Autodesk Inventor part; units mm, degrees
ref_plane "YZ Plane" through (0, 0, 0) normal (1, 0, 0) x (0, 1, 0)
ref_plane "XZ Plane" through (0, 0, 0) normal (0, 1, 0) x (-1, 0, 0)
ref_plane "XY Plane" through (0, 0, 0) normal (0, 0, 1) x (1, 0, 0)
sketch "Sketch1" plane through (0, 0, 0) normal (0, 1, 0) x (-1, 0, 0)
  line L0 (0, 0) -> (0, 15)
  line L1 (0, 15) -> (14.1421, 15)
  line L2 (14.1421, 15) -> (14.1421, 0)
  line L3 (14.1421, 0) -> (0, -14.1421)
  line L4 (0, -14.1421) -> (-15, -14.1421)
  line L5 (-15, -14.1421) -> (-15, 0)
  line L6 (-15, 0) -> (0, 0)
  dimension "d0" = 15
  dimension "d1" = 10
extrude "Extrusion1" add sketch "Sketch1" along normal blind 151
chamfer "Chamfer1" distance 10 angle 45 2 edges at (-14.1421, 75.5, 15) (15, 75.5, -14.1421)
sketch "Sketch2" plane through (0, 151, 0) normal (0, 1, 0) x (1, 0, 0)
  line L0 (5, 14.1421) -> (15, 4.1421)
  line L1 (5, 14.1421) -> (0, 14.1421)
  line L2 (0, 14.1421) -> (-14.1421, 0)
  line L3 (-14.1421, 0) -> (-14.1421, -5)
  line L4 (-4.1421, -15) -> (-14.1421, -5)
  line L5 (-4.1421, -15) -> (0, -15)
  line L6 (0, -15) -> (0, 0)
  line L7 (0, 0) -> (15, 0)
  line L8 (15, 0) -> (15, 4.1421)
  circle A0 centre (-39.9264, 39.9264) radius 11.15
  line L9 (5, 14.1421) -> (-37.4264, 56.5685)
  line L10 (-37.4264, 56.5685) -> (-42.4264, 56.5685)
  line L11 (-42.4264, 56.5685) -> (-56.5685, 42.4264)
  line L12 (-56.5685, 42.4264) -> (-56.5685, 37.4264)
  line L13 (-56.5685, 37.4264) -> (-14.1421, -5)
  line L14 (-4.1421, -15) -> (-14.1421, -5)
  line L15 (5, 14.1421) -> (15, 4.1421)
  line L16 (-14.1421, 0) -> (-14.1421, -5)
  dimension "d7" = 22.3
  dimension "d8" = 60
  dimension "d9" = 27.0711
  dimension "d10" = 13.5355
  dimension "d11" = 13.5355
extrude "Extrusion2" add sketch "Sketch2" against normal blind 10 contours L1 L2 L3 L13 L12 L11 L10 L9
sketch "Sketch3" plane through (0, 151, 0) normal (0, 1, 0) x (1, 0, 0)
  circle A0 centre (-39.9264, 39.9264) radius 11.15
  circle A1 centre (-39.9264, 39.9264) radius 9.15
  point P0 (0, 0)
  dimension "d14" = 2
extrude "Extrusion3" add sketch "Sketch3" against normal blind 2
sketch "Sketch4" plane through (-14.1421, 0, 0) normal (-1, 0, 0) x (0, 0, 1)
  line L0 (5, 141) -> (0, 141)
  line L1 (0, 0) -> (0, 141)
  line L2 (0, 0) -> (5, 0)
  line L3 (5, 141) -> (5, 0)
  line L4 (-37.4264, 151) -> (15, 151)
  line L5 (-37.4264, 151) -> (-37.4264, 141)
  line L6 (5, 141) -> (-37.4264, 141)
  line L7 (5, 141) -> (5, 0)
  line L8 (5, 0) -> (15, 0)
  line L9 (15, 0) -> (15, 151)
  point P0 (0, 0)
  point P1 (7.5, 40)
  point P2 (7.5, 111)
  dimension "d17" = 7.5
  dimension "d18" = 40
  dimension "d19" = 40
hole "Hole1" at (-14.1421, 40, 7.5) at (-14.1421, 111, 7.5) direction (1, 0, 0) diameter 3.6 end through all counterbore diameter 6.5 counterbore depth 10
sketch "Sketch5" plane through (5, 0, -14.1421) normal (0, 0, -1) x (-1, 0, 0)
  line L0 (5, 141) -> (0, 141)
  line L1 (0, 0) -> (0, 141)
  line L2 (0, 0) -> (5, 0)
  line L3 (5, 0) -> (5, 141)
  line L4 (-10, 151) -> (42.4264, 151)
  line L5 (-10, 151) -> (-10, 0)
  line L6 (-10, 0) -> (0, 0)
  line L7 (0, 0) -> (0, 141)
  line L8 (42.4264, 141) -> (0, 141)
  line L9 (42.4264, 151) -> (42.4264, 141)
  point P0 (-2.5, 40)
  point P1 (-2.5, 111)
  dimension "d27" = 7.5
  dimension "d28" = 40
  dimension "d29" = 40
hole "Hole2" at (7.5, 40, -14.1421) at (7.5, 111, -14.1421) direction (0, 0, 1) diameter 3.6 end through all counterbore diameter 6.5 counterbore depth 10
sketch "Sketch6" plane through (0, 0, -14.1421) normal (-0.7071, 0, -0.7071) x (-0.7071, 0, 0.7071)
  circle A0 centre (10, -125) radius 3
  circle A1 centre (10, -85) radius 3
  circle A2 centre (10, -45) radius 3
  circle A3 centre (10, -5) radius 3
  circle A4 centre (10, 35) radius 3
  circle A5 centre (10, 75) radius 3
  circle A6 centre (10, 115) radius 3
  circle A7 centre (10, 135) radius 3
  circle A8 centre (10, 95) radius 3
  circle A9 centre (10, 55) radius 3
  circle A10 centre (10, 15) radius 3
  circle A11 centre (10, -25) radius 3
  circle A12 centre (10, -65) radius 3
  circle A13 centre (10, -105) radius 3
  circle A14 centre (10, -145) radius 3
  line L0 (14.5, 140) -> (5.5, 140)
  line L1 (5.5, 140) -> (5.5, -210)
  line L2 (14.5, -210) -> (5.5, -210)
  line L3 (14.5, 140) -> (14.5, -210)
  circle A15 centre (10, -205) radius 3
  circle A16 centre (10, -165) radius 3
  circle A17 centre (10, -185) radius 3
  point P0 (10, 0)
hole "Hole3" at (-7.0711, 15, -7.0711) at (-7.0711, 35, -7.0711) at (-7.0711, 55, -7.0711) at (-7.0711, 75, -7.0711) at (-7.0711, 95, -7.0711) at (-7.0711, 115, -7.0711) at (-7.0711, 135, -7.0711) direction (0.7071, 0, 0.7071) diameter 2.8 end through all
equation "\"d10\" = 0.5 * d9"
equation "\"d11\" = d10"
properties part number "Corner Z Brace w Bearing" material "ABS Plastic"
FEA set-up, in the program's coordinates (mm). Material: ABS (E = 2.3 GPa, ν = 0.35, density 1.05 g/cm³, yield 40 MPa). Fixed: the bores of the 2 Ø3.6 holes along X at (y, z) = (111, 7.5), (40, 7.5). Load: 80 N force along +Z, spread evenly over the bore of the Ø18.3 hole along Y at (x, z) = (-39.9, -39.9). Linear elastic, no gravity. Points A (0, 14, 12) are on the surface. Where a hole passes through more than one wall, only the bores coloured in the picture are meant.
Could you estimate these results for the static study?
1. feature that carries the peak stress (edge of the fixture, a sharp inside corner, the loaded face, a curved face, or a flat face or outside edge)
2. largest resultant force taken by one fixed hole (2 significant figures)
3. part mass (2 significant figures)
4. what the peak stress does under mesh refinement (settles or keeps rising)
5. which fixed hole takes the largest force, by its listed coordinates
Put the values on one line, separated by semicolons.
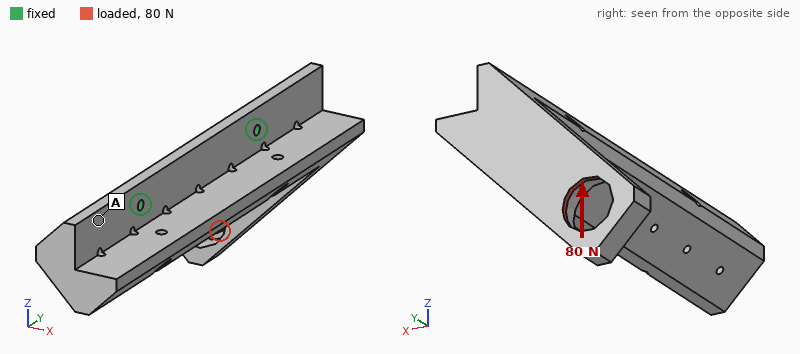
edge of the fixture; 150 N; 79 g; keeps rising; (111, 7.5)
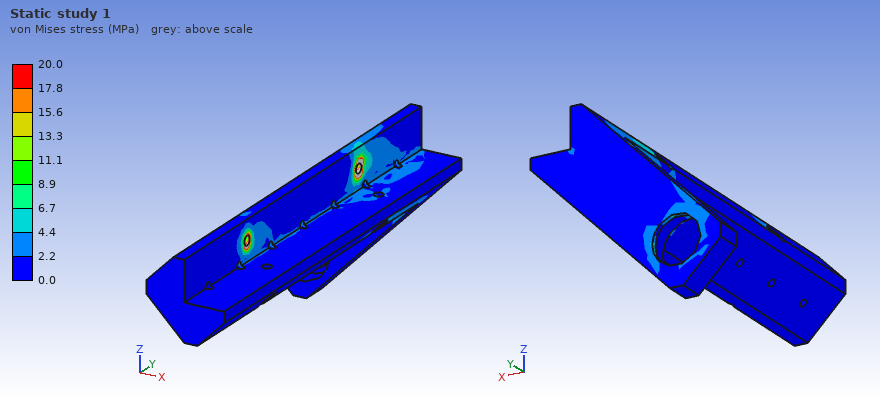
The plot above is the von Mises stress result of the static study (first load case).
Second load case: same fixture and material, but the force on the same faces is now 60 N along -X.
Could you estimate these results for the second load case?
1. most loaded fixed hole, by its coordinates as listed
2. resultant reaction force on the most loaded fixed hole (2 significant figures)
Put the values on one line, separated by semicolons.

(111, 7.5); 92 N
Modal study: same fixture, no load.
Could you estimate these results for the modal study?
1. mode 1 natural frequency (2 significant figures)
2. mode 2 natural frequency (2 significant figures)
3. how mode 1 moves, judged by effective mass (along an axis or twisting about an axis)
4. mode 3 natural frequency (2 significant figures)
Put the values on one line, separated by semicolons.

330 Hz; 500 Hz; along X; 940 Hz
